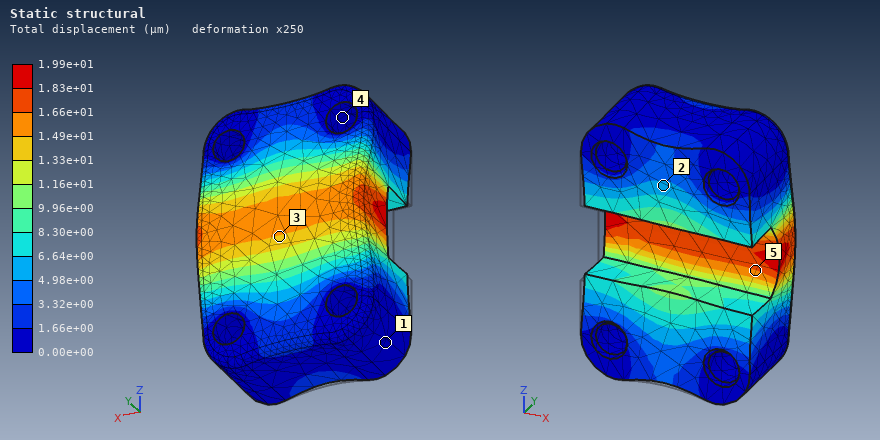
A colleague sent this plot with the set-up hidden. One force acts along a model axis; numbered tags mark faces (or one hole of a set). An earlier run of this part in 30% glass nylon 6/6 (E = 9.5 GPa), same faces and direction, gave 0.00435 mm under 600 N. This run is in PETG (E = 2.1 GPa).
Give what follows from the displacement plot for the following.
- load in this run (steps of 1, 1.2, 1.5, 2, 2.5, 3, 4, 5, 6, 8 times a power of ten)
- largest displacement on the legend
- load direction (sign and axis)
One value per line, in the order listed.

600 N
1.99e+01 µm
+Y
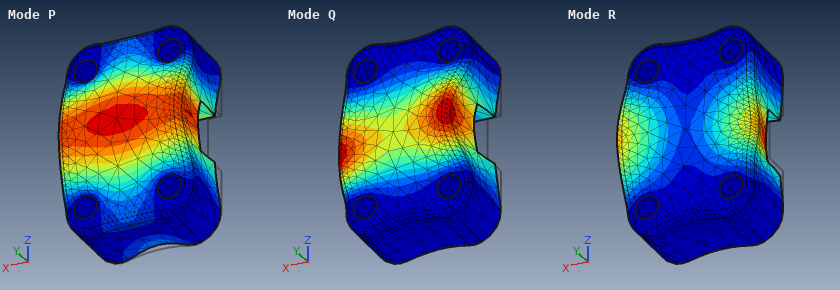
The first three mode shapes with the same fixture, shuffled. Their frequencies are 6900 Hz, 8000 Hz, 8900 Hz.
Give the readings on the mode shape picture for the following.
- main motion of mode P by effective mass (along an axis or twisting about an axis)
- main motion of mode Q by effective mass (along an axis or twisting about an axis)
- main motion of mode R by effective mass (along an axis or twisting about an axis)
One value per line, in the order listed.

along Y
along X
along X
